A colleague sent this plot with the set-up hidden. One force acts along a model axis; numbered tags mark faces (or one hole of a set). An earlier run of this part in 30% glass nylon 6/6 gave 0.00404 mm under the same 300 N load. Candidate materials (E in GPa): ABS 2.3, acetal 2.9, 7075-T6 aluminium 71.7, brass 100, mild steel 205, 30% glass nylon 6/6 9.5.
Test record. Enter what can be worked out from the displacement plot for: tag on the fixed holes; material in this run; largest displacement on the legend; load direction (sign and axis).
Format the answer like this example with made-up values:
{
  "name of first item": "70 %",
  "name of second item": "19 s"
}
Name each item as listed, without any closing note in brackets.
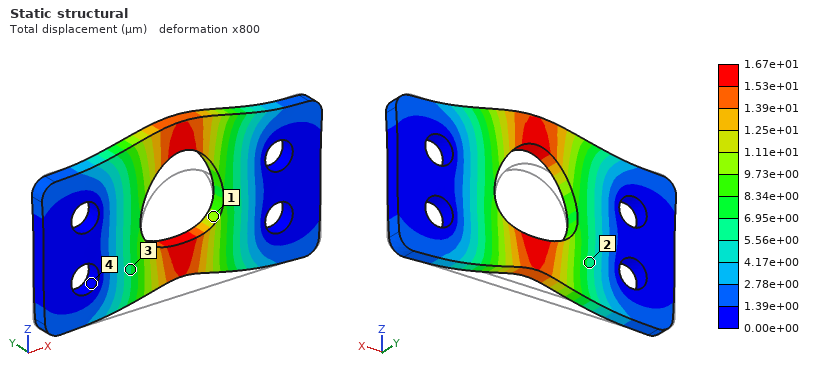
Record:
{
  "tag on the fixed holes": "4",
  "material in this run": "ABS",
  "largest displacement on the legend": "1.67e+01 µm",
  "load direction": "+Z"
}
